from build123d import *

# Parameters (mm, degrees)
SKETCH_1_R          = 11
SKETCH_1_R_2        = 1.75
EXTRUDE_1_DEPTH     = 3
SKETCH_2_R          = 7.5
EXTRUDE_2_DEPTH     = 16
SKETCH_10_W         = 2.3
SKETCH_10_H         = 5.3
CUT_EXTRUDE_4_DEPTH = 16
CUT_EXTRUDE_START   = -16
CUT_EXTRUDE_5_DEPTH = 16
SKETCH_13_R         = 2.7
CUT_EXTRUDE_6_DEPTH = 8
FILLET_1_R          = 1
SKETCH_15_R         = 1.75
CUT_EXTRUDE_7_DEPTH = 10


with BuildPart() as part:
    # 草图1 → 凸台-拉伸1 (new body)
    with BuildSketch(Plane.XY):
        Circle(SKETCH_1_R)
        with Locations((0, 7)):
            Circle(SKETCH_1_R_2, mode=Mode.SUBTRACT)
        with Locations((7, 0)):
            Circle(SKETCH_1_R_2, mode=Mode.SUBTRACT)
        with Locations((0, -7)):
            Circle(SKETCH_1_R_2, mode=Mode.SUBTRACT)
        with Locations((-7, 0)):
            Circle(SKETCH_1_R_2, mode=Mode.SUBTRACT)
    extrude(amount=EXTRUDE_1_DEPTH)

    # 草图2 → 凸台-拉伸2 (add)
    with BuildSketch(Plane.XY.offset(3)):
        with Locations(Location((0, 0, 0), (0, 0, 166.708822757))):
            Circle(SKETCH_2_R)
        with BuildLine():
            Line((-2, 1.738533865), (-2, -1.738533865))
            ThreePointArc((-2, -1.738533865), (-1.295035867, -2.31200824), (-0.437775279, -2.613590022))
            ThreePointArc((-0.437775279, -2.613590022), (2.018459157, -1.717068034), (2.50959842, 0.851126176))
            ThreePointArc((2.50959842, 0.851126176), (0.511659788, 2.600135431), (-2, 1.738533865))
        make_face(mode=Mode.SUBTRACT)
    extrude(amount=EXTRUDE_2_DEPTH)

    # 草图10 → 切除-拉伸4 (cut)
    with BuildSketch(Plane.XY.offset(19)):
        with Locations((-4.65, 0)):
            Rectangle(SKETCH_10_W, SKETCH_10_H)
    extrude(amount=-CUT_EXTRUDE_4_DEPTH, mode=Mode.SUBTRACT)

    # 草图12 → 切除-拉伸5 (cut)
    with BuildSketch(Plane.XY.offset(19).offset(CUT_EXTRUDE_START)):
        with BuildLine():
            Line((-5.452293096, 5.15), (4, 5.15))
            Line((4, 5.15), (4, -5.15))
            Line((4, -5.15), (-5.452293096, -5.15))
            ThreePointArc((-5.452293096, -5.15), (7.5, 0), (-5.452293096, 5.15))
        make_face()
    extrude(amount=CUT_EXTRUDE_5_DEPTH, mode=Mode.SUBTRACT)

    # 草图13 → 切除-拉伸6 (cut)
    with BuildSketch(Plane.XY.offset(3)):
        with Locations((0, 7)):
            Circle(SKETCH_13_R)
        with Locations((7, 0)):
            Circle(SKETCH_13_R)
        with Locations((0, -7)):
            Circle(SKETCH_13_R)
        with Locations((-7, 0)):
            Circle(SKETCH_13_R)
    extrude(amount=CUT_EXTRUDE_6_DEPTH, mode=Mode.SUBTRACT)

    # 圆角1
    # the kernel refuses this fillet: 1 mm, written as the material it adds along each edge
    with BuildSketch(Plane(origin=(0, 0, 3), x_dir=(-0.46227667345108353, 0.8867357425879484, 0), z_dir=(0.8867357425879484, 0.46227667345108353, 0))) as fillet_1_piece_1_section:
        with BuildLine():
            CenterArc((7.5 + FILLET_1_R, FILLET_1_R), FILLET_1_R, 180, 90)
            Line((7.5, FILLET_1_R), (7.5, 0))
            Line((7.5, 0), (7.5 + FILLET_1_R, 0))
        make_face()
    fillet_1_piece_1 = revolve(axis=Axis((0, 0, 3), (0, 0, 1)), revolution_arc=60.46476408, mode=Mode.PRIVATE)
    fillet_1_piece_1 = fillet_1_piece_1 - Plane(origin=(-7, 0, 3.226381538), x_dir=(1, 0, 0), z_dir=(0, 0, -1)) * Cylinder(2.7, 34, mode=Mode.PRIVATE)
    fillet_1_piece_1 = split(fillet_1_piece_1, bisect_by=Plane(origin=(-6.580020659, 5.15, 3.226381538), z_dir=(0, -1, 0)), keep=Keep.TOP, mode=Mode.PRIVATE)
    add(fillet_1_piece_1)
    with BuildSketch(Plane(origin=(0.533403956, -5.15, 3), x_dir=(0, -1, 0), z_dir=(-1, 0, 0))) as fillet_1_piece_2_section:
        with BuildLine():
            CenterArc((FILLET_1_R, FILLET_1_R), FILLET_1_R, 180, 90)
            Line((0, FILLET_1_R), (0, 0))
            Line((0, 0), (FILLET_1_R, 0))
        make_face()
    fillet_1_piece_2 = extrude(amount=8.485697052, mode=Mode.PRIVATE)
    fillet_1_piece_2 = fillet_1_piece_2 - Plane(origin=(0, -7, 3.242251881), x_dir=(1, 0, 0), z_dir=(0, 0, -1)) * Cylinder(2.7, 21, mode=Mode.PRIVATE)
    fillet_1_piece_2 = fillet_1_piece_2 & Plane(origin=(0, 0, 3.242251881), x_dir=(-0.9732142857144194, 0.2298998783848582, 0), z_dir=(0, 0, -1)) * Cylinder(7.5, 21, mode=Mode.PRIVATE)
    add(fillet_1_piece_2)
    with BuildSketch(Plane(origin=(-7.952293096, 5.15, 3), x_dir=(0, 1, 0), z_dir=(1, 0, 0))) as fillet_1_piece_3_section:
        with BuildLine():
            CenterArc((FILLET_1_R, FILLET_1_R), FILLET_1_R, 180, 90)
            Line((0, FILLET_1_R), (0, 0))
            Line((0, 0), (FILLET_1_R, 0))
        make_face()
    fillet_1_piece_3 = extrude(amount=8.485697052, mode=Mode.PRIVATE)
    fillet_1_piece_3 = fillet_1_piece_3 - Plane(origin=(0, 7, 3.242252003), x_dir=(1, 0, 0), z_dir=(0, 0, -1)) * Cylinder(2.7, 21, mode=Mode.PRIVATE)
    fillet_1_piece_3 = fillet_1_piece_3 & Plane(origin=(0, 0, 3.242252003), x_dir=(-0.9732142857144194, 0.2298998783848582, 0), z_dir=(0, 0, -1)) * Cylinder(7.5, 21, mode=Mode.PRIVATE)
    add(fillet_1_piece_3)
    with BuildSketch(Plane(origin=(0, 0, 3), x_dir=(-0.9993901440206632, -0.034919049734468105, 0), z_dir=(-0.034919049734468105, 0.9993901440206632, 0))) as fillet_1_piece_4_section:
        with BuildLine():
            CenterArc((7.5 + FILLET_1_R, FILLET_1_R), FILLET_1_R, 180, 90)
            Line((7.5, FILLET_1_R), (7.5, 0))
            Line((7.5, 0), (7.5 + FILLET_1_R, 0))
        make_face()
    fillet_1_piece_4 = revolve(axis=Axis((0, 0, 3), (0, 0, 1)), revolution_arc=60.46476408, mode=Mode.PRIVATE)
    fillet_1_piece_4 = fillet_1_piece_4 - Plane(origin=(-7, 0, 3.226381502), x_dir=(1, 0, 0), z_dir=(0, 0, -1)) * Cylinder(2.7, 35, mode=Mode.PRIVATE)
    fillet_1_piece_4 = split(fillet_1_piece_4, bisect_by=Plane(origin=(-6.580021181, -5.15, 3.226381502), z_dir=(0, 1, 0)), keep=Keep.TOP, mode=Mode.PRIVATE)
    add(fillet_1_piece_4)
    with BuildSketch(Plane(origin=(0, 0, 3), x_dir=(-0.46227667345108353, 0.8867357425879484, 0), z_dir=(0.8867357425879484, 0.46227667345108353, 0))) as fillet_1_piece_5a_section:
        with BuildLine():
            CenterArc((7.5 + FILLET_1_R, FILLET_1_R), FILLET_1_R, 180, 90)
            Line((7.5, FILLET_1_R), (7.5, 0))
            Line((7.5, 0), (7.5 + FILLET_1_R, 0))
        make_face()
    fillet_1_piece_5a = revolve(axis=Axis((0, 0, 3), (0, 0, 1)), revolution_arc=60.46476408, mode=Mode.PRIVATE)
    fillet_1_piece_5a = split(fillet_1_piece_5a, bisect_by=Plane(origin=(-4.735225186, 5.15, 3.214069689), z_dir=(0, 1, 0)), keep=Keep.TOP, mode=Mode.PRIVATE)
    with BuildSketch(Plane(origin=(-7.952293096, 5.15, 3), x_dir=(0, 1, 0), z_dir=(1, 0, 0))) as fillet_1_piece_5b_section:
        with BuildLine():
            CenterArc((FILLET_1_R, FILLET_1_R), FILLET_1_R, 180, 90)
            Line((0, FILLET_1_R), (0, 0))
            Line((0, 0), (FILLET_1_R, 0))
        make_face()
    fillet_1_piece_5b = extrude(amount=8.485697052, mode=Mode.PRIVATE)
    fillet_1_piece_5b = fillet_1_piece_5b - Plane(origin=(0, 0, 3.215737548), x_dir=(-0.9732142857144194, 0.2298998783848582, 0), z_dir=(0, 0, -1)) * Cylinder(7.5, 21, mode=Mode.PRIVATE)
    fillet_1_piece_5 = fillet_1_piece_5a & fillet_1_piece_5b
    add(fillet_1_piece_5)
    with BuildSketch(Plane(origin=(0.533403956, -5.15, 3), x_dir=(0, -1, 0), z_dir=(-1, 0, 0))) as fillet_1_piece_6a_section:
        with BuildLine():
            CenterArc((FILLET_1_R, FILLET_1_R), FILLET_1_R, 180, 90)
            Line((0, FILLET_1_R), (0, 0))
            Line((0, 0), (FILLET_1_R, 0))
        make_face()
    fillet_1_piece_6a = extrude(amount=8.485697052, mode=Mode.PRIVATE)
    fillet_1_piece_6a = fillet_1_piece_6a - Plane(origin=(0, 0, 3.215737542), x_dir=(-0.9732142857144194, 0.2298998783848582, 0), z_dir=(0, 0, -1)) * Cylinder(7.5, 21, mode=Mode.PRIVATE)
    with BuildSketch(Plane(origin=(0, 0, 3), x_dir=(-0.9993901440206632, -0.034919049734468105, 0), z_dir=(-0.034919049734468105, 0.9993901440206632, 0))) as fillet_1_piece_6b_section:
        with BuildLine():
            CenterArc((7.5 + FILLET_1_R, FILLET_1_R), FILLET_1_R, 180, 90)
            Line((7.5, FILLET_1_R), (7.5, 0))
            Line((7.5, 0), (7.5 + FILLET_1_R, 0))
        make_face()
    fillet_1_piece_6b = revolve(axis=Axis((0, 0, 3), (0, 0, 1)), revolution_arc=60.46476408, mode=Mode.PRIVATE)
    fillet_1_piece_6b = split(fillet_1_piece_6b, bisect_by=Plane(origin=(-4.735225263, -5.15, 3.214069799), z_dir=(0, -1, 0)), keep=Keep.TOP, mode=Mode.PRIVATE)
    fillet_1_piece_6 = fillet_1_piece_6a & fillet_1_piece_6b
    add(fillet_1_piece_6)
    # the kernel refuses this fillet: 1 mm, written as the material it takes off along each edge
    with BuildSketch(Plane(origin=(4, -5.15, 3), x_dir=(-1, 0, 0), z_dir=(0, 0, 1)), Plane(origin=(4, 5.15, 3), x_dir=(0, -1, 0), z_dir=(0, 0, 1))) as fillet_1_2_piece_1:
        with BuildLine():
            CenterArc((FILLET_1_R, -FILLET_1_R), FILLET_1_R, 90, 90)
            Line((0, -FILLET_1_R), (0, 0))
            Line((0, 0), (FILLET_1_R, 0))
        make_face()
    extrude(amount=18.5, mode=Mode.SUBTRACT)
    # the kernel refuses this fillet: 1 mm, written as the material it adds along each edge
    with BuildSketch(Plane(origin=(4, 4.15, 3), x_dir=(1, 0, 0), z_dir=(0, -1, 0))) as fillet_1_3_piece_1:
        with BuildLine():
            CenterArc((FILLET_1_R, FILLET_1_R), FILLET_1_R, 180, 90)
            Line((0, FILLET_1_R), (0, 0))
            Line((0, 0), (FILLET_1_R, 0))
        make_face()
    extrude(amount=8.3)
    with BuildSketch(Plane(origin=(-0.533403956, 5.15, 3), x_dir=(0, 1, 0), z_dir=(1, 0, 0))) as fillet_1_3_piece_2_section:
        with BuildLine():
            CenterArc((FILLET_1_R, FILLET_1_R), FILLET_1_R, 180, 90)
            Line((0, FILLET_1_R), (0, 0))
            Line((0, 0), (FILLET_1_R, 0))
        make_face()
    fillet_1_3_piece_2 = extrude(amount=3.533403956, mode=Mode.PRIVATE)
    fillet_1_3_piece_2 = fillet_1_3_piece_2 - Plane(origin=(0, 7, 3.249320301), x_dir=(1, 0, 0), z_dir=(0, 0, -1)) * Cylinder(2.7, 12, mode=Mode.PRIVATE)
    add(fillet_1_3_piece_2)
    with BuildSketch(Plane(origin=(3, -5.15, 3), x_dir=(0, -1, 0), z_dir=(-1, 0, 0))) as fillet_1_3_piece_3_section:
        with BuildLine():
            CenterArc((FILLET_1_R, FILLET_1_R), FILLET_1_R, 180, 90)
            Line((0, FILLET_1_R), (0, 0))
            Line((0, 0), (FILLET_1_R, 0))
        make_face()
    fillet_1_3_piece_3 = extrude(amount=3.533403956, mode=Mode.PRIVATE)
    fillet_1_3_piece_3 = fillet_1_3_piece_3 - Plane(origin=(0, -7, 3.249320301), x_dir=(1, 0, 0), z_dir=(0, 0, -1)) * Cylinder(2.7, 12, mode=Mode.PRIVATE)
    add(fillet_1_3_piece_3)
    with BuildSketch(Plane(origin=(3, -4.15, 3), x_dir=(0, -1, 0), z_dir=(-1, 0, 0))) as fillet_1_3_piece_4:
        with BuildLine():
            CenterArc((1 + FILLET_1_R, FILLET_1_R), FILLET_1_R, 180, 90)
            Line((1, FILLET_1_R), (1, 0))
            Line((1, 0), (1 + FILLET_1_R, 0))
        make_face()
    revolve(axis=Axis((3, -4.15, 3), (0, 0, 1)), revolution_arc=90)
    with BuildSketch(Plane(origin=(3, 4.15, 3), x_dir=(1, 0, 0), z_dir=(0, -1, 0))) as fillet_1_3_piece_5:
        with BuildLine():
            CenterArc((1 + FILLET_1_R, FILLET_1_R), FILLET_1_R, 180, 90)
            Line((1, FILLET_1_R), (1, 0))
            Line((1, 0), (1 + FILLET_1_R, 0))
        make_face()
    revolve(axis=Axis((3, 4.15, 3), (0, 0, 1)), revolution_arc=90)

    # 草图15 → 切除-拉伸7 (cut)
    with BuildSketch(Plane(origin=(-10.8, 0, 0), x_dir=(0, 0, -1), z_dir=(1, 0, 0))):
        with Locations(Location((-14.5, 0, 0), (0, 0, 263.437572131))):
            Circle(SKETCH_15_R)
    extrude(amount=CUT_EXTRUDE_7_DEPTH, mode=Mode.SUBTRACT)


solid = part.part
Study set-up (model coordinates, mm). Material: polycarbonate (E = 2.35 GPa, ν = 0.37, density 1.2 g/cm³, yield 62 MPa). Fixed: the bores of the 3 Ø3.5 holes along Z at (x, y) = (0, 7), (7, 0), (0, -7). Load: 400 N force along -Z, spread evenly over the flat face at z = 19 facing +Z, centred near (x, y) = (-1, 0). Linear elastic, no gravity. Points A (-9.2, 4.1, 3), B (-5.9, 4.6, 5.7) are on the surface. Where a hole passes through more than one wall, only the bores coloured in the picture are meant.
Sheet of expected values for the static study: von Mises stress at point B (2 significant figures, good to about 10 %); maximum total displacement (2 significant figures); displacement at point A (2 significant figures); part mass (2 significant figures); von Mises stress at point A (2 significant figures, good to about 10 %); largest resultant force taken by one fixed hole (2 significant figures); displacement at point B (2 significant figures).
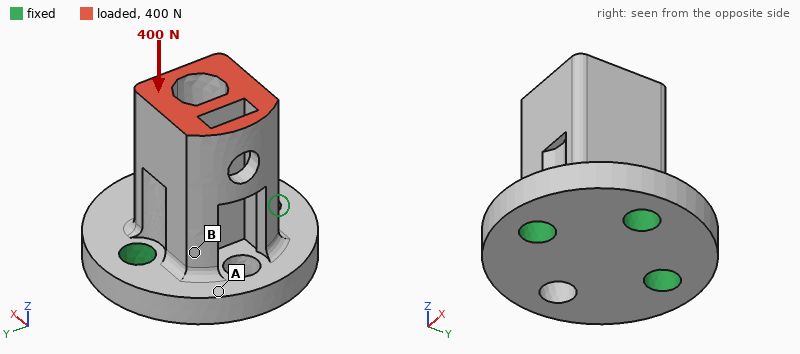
8.8 MPa
0.20 mm
0.10 mm
2.6 g
2.5 MPa
190 N
0.086 mm
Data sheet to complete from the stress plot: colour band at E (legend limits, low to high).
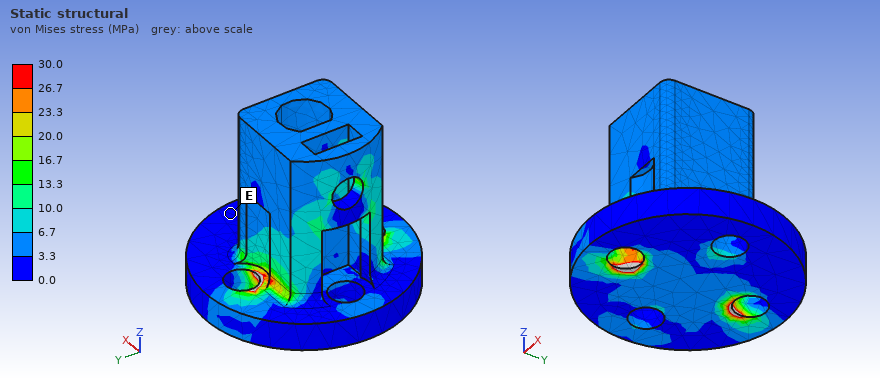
0.0 to 3.3 MPa
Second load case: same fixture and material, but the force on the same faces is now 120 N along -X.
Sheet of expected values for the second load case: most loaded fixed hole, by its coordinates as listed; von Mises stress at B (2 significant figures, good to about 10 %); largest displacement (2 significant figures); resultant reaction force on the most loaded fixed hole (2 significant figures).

(7, 0)
13 MPa
0.41 mm
190 N
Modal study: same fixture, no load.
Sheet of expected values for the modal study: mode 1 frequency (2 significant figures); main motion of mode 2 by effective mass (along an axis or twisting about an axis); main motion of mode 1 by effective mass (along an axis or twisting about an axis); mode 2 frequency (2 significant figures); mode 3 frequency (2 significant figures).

3900 Hz
along Y
along X
5200 Hz
8800 Hz
